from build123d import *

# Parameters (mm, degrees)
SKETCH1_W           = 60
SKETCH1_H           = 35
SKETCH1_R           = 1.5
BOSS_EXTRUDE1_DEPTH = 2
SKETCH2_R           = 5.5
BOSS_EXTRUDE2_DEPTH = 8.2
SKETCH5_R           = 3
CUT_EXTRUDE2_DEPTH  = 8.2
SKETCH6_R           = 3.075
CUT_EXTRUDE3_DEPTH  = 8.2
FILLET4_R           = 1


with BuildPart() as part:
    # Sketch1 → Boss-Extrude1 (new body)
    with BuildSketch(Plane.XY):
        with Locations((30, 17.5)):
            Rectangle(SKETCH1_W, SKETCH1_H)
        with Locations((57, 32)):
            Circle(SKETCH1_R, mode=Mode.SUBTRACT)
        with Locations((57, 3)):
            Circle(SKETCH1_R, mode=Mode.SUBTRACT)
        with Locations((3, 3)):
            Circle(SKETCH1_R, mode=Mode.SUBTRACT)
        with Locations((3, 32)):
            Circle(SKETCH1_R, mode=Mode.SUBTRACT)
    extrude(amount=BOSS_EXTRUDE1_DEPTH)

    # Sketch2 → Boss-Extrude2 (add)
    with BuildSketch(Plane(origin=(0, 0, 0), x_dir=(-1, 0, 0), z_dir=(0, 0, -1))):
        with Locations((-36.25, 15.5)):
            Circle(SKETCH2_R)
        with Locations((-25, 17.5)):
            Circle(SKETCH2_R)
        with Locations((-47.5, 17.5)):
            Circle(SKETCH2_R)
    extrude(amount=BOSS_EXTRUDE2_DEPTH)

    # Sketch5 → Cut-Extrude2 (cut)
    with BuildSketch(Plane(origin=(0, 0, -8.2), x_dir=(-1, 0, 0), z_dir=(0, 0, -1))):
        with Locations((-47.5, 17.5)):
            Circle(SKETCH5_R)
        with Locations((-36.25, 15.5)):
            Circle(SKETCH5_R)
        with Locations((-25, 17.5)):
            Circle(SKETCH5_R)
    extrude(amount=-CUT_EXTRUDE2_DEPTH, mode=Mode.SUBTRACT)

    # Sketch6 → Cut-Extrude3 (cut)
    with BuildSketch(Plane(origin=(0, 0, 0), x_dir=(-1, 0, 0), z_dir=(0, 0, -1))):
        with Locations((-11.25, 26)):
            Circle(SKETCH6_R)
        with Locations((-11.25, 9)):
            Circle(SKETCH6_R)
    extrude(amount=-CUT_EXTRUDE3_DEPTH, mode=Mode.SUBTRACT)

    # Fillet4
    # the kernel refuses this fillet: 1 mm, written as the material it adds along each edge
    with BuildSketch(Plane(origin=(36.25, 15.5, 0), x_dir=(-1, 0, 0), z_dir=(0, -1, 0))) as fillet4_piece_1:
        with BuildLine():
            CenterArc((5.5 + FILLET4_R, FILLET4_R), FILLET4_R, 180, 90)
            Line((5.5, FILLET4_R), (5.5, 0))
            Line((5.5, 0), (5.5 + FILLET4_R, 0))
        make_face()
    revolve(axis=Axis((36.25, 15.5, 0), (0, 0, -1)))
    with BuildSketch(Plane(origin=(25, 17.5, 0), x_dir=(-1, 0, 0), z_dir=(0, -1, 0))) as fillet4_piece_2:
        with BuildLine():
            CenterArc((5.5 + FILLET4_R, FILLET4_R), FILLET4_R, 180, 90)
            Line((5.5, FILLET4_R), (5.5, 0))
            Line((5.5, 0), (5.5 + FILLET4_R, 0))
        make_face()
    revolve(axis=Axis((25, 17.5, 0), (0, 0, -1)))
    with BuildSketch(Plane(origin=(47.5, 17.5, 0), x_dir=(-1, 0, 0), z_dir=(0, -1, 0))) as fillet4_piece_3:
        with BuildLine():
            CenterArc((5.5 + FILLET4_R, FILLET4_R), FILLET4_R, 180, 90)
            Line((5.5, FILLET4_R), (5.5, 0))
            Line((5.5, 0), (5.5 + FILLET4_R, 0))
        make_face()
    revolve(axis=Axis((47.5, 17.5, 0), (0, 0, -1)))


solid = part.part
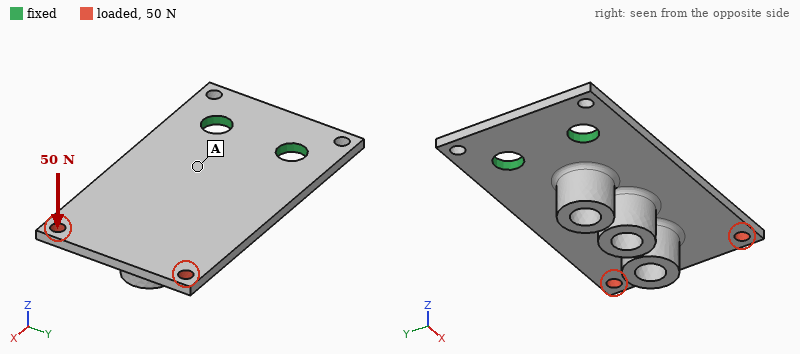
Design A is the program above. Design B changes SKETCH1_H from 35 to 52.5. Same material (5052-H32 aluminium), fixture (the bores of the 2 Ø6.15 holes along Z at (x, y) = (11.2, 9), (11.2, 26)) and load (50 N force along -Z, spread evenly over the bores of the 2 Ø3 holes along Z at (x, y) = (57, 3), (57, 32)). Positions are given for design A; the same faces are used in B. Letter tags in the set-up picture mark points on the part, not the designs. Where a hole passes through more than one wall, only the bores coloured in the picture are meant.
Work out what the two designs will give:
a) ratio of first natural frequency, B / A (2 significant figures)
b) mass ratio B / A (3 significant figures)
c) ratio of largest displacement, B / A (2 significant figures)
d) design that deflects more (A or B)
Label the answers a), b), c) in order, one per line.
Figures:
a) 0.96
b) 1.37
c) 0.78
d) A
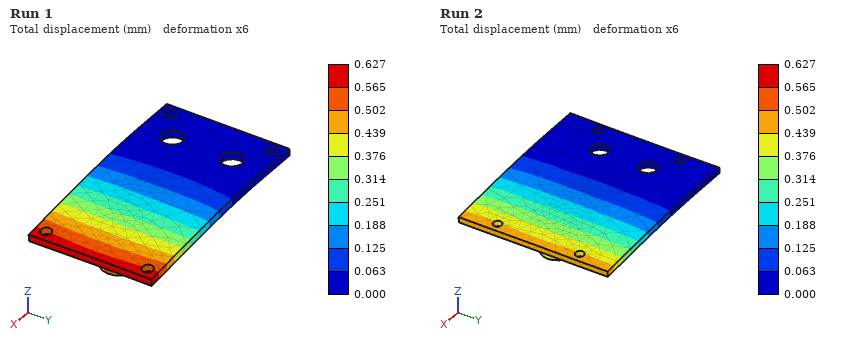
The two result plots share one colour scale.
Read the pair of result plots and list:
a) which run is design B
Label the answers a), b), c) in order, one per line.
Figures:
a) Run 2
